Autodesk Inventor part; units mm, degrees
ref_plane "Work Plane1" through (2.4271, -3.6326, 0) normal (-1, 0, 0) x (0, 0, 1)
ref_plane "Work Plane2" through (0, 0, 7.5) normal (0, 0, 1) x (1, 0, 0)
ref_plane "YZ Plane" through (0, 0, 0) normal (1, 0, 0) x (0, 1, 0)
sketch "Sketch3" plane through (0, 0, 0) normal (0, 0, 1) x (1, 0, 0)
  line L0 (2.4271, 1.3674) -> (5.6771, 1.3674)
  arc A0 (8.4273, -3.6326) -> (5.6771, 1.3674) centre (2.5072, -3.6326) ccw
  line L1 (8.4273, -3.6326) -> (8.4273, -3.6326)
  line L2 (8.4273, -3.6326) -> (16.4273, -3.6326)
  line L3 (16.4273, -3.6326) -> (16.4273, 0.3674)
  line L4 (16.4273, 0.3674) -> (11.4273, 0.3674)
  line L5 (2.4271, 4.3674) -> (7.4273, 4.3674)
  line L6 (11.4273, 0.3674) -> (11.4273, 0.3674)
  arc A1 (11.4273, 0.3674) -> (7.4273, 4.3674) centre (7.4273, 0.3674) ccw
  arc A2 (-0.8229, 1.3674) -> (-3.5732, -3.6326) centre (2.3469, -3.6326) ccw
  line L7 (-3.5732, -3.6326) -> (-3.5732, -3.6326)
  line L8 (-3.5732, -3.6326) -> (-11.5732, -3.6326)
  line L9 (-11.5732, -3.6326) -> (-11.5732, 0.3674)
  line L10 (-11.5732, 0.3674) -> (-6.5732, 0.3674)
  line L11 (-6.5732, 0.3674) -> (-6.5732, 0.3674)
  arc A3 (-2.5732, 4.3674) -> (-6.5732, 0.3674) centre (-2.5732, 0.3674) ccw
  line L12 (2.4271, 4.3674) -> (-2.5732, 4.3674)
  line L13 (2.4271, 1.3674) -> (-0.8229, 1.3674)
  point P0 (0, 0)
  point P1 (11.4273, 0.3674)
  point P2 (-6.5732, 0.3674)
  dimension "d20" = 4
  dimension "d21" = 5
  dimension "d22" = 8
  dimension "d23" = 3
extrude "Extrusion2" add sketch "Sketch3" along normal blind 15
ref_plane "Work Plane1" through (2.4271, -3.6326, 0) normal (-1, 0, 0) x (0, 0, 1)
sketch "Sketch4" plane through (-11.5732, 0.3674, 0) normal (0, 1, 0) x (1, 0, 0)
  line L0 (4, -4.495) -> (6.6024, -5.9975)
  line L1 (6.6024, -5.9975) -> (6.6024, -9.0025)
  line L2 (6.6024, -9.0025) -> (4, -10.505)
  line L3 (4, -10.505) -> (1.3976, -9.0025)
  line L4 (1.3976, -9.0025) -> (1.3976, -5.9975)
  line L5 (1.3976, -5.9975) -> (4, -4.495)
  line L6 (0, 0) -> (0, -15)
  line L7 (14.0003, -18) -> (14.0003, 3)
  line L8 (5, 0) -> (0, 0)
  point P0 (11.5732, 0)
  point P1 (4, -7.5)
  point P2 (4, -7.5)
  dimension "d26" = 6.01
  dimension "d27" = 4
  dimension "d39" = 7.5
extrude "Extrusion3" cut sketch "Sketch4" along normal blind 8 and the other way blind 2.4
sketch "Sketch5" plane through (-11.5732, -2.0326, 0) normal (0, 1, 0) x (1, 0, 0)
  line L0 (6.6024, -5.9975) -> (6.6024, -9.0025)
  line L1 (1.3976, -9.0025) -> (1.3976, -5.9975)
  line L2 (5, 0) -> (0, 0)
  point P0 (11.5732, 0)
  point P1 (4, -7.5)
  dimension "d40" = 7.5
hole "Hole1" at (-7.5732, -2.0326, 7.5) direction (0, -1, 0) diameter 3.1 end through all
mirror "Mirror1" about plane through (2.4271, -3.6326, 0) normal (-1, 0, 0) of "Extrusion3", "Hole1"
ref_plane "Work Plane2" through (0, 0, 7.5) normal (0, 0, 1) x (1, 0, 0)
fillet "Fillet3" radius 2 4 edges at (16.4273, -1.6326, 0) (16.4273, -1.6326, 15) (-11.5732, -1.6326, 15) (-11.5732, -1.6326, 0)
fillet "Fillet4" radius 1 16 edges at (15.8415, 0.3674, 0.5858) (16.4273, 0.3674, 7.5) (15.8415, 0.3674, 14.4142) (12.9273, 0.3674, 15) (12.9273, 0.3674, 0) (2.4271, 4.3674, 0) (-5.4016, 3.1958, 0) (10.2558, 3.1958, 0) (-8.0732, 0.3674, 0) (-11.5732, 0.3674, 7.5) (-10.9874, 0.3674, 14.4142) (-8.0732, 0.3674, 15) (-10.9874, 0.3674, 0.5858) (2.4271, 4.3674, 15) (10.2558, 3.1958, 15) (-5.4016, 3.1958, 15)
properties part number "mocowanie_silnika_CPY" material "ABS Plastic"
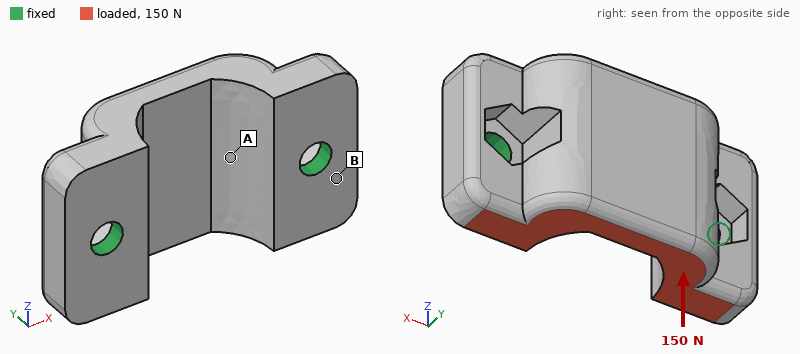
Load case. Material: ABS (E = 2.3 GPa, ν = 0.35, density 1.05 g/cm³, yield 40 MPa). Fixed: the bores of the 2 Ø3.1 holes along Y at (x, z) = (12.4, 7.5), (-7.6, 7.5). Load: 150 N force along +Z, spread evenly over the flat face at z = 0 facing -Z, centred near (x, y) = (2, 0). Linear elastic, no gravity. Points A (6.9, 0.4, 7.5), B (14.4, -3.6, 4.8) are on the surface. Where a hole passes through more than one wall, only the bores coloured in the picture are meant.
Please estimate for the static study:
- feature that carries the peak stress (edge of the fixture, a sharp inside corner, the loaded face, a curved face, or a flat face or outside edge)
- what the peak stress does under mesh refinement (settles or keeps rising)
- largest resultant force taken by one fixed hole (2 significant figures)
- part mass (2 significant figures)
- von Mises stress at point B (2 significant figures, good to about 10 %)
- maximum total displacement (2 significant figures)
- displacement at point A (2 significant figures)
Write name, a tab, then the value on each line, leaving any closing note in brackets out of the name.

feature that carries the peak stress	edge of the fixture
what the peak stress does under mesh refinement	keeps rising
largest resultant force taken by one fixed hole	75 N
part mass	1.8 g
von Mises stress at point B	5.4 MPa
maximum total displacement	0.15 mm
displacement at point A	0.058 mm
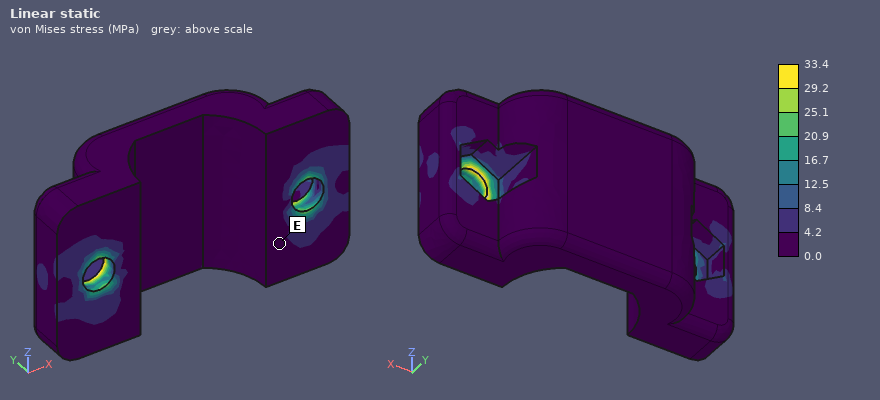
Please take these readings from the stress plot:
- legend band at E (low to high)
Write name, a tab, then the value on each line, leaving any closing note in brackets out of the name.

legend band at E	0.0 to 4.2 MPa
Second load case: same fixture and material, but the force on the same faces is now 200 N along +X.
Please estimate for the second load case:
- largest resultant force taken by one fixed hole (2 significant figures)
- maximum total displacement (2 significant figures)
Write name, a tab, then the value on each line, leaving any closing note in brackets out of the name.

largest resultant force taken by one fixed hole	110 N
maximum total displacement	0.10 mm
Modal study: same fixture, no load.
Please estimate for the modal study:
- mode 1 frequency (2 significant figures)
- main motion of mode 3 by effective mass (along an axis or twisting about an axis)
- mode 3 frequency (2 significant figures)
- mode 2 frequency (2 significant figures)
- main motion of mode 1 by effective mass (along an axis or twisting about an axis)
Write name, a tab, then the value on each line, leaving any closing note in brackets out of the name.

mode 1 frequency	3700 Hz
main motion of mode 3 by effective mass	along X
mode 3 frequency	10 kHz
mode 2 frequency	8400 Hz
main motion of mode 1 by effective mass	along Z
